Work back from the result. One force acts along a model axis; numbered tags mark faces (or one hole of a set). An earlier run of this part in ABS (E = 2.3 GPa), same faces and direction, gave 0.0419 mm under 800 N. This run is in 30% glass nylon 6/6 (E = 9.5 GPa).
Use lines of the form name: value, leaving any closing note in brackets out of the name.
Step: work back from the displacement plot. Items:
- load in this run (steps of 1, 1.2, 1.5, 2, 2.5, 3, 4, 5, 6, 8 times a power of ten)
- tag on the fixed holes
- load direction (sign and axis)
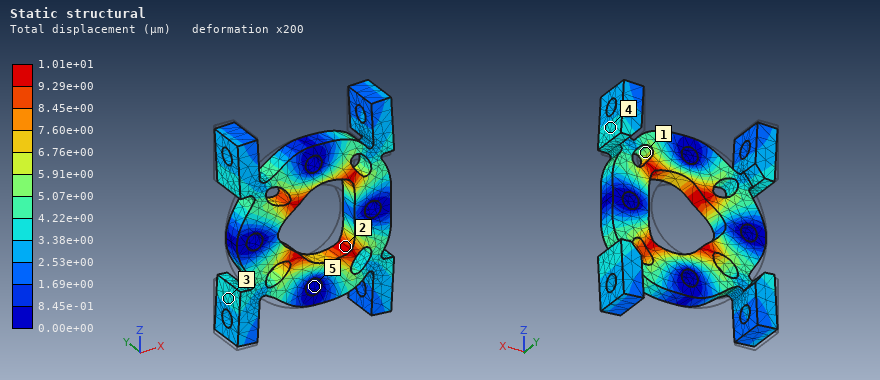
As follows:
load in this run: 800 N
tag on the fixed holes: 5
load direction: +X
